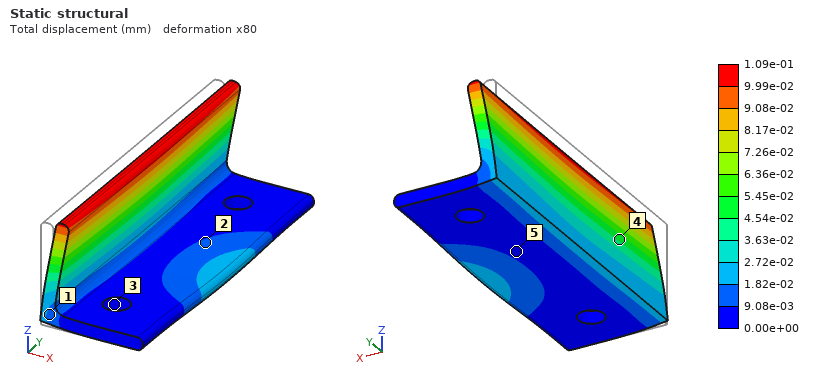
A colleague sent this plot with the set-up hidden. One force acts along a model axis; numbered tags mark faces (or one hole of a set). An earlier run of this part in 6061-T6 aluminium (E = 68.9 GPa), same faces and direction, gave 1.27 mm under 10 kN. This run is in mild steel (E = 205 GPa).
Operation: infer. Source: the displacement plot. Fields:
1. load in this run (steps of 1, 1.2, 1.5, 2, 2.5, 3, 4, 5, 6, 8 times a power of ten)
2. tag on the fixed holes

2.5 kN
3
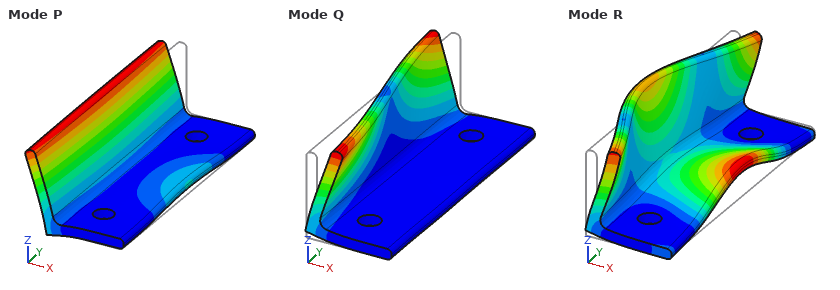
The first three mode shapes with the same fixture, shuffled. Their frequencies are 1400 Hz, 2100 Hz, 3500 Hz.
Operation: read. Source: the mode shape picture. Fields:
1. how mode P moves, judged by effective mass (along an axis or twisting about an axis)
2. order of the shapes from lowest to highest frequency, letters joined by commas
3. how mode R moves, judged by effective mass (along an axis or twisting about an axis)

along X
P, Q, R
along Z
